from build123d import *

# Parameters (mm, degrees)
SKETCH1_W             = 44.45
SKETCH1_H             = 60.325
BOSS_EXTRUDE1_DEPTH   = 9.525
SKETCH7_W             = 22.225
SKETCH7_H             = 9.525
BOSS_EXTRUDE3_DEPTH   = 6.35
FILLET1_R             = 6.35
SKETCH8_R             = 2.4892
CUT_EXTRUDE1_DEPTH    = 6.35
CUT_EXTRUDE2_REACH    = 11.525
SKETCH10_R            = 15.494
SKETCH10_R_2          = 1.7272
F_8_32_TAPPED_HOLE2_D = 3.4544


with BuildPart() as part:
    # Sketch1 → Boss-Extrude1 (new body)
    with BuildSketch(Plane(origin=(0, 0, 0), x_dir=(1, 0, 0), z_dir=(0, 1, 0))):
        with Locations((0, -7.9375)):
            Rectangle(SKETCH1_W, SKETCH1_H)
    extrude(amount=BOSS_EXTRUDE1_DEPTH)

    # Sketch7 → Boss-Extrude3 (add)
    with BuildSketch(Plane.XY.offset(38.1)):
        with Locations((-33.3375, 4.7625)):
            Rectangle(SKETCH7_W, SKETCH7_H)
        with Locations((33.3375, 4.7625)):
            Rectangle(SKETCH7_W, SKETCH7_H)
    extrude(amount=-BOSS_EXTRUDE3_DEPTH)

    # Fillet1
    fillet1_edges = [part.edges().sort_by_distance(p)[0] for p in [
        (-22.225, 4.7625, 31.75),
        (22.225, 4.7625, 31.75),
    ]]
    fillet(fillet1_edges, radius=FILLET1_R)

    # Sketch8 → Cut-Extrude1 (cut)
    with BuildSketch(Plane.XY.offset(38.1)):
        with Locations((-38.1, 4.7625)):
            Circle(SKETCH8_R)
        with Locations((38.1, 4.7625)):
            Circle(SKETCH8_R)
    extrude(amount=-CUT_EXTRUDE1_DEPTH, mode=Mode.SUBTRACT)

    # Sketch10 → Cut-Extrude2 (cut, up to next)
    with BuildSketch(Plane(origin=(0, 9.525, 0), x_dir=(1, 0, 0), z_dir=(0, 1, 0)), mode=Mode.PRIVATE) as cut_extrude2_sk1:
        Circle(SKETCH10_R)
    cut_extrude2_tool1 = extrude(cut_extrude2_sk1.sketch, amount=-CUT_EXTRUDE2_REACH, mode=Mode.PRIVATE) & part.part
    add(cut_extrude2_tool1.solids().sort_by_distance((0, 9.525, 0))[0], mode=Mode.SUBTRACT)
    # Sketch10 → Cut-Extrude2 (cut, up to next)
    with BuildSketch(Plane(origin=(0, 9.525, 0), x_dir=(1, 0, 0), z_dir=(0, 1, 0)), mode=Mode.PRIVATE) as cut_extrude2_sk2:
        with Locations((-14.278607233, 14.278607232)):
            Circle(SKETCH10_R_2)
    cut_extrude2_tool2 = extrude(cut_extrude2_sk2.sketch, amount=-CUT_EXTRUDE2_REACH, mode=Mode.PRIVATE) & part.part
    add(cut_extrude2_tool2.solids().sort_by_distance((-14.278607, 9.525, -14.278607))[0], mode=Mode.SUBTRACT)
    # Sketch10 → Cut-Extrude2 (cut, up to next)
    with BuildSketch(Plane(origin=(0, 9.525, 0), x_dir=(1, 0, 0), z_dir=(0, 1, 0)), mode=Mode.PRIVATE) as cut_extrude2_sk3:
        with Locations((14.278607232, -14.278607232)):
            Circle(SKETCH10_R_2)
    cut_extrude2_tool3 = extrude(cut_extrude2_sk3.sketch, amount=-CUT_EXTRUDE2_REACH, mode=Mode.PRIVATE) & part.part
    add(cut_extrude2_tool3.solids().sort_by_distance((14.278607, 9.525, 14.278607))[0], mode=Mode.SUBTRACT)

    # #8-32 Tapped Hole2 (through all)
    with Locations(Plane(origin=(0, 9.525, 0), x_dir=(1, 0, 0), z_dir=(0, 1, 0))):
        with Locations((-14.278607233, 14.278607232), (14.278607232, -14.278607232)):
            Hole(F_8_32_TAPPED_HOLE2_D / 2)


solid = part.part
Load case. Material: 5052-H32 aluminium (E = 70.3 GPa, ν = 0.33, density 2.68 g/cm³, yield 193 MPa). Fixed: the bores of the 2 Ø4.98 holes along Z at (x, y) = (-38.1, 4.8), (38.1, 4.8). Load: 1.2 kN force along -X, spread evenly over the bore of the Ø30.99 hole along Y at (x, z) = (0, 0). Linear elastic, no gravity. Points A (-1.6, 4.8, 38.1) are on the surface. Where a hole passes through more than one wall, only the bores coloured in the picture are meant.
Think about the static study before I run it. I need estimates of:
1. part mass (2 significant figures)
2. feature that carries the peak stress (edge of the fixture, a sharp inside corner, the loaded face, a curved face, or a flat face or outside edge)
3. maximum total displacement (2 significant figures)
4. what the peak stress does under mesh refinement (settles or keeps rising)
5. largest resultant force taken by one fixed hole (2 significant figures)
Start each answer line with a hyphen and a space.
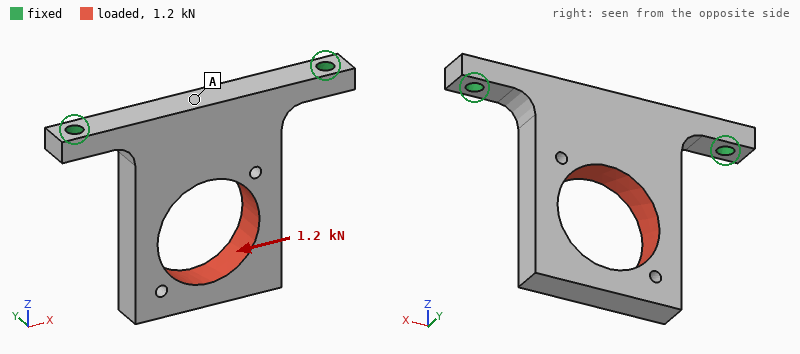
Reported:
- 56 g
- edge of the fixture
- 74 µm
- keeps rising
- 910 N
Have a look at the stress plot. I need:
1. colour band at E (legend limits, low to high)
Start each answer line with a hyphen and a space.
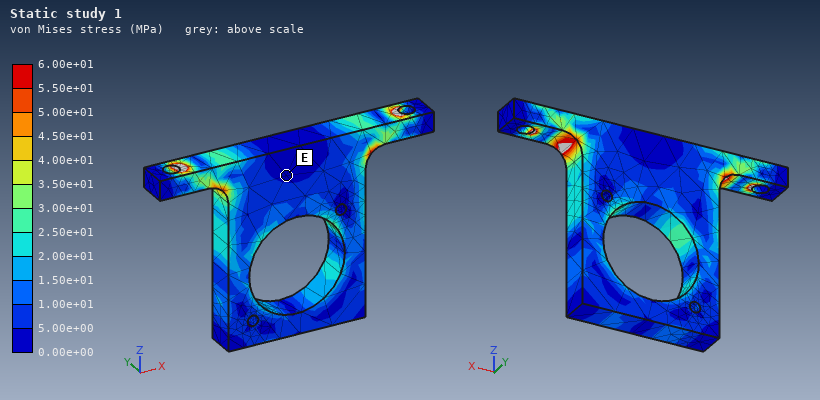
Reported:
- 0.00e+00 to 5.00e+00 MPa
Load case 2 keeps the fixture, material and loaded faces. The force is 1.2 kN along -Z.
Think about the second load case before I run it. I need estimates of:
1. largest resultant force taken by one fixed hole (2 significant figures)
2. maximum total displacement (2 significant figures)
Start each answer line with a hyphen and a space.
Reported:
- 730 N
- 25 µm
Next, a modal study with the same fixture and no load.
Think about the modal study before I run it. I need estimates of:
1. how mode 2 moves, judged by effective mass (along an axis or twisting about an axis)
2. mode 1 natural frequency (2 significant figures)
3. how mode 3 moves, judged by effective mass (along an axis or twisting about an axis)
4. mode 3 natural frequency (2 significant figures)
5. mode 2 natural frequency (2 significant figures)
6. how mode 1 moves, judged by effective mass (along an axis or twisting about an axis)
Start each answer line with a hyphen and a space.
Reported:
- along X
- 940 Hz
- twisting about Z
- 4300 Hz
- 4100 Hz
- along Y
